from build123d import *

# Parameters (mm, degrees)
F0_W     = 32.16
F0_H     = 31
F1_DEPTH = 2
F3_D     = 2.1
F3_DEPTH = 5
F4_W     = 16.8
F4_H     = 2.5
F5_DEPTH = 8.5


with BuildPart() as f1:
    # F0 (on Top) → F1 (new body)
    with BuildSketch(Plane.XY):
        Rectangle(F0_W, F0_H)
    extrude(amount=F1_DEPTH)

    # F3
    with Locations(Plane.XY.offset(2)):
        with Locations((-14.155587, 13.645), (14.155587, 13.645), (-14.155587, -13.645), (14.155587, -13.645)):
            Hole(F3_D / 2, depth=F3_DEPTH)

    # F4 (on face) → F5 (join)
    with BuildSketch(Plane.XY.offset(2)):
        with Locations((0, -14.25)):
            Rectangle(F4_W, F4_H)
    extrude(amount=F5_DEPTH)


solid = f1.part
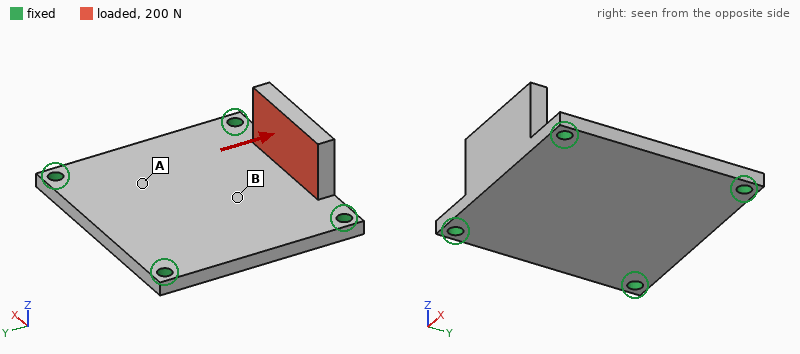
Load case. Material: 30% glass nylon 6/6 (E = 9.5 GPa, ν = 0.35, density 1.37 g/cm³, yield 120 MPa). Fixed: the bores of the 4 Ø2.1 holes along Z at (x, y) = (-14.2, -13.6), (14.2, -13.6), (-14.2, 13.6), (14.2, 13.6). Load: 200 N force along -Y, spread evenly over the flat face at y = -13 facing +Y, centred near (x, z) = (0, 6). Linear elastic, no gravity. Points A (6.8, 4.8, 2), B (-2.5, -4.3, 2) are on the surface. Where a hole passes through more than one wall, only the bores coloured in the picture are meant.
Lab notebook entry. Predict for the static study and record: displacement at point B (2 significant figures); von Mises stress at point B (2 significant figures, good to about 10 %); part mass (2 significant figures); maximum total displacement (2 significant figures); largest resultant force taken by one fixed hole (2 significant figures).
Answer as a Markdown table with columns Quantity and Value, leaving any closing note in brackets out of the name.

| Quantity | Value |
|---|---|
| displacement at point B | 0.10 mm |
| von Mises stress at point B | 21 MPa |
| part mass | 3.2 g |
| maximum total displacement | 0.45 mm |
| largest resultant force taken by one fixed hole | 67 N |
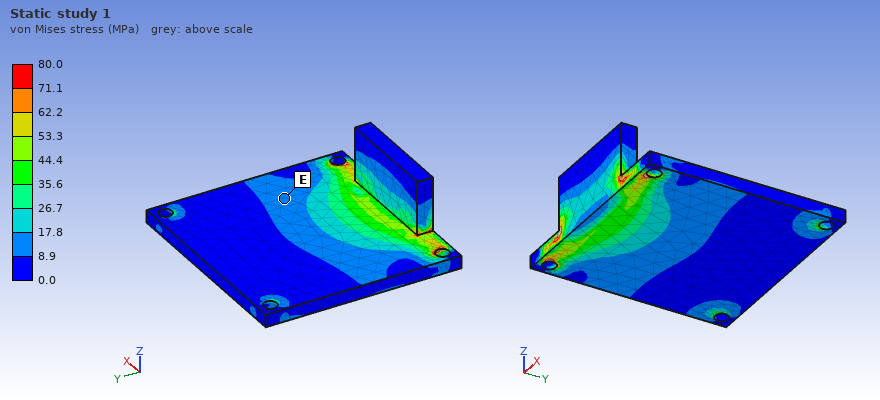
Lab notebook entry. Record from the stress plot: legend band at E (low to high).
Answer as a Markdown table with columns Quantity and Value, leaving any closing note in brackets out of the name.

| Quantity | Value |
|---|---|
| legend band at E | 8.9 to 17.8 MPa |
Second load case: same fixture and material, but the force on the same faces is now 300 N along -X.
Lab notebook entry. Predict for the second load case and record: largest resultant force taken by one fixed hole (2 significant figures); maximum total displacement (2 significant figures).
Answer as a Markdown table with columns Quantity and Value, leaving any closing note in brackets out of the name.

| Quantity | Value |
|---|---|
| largest resultant force taken by one fixed hole | 150 N |
| maximum total displacement | 0.12 mm |
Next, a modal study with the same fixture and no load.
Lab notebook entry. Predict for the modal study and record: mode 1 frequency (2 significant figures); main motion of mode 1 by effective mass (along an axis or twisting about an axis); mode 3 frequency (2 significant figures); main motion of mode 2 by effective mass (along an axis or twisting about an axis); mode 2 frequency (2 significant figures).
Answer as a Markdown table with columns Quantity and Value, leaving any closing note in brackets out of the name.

| Quantity | Value |
|---|---|
| mode 1 frequency | 4400 Hz |
| main motion of mode 1 by effective mass | along Z |
| mode 3 frequency | 7900 Hz |
| main motion of mode 2 by effective mass | along Z |
| mode 2 frequency | 6200 Hz |
